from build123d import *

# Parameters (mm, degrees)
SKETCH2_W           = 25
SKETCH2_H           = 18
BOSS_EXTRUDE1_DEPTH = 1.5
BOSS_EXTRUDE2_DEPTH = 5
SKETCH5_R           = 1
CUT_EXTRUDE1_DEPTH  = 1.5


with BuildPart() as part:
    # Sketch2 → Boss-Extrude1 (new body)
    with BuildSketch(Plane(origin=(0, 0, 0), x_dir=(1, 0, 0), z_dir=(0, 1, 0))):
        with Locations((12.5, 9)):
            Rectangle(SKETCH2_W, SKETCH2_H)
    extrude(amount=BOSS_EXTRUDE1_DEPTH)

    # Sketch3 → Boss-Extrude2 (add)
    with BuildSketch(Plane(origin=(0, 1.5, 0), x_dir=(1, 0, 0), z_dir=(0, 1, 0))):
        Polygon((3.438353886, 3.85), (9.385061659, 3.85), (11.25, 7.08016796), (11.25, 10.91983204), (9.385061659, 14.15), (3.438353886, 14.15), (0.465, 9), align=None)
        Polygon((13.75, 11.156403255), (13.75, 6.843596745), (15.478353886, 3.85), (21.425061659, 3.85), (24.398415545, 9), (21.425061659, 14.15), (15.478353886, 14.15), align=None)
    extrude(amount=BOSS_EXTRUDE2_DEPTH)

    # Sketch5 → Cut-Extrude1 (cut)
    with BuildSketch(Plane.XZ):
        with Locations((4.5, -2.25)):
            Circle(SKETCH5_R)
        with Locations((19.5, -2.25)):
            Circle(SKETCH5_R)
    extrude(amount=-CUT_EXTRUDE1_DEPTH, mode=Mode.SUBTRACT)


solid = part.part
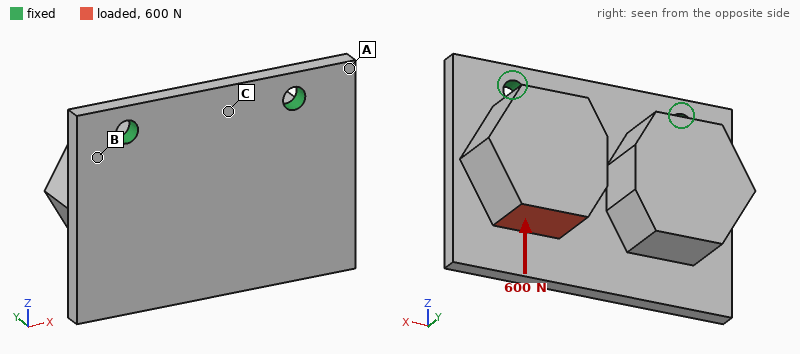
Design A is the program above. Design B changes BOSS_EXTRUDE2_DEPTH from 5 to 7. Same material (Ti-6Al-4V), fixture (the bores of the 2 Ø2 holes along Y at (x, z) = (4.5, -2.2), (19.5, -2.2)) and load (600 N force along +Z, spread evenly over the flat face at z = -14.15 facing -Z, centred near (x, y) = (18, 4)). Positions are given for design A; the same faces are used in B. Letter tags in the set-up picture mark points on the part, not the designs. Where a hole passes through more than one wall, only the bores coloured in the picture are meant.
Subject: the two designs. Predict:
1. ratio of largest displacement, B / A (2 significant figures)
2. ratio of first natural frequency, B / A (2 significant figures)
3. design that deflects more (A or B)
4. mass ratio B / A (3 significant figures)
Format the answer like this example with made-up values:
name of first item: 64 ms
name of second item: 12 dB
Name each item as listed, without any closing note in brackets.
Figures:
ratio of largest displacement, B / A: 1.3
ratio of first natural frequency, B / A: 0.86
design that deflects more: B
mass ratio B / A: 1.23
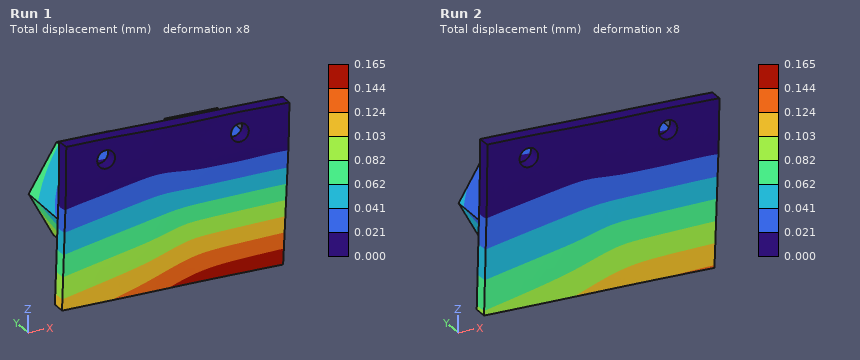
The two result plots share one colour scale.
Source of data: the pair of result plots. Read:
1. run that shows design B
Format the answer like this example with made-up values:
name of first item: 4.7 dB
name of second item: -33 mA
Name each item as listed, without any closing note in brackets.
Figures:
run that shows design B: Run 1
